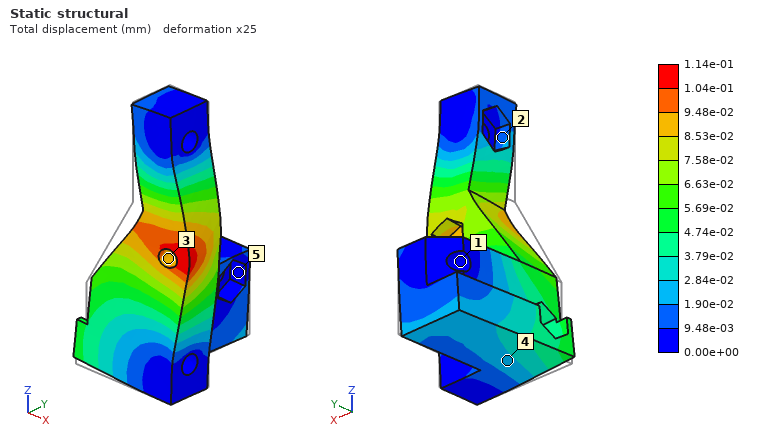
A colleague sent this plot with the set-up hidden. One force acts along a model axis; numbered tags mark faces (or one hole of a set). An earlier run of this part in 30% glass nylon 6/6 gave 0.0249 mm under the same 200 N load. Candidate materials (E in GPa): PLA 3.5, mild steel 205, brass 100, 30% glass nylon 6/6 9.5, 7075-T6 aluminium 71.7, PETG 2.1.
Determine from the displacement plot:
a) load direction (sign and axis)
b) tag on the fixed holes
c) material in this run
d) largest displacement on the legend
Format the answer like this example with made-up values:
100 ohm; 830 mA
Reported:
+X; 1; PETG; 1.14e-01 mm
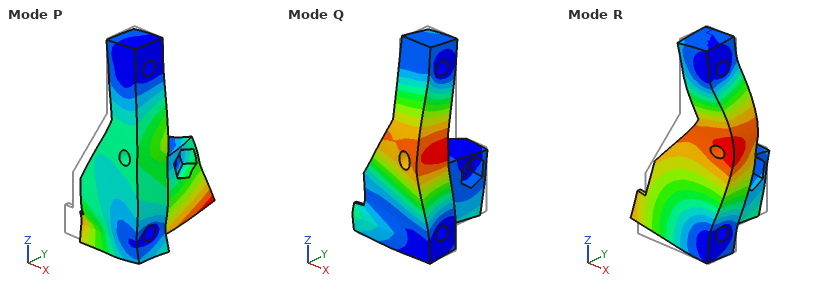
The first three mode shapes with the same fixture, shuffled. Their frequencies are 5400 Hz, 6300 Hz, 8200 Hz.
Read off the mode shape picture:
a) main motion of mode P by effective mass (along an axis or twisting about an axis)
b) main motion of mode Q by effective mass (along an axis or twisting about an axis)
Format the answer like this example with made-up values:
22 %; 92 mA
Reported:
along X; along Y
